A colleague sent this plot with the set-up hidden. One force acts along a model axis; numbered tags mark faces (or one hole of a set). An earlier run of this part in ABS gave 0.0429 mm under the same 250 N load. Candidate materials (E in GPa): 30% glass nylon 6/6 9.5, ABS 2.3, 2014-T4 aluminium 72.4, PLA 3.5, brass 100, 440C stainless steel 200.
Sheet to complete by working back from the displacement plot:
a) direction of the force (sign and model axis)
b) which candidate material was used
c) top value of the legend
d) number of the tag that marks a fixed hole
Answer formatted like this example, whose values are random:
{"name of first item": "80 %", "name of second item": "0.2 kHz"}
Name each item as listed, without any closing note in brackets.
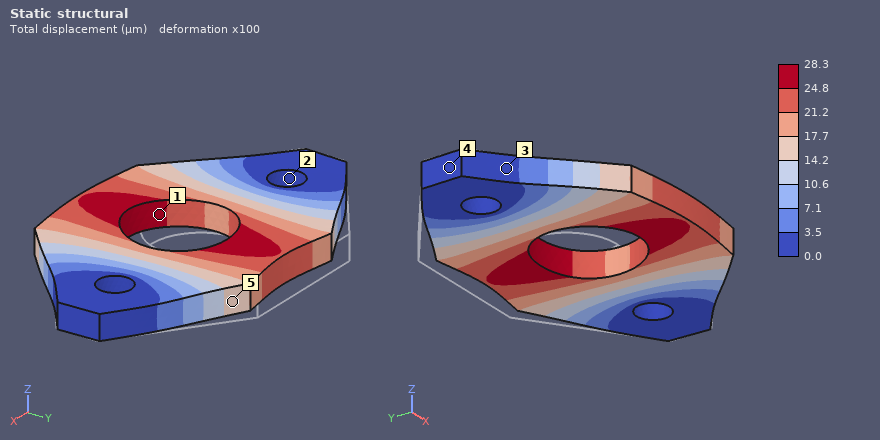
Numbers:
{"direction of the force": "-Y", "which candidate material was used": "PLA", "top value of the legend": "28.3 µm", "number of the tag that marks a fixed hole": "2"}
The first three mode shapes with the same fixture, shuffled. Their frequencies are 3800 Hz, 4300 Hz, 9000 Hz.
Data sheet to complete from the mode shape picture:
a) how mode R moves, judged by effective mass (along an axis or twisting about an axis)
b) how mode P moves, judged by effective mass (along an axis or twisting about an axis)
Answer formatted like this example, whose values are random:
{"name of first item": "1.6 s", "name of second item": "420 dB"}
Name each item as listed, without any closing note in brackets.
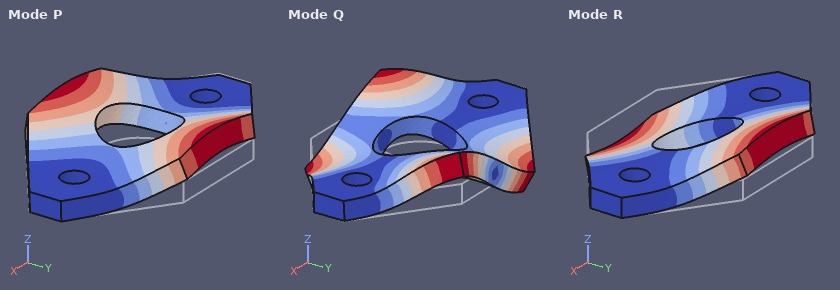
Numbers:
{"how mode R moves, judged by effective mass": "twisting about X", "how mode P moves, judged by effective mass": "along Z"}
